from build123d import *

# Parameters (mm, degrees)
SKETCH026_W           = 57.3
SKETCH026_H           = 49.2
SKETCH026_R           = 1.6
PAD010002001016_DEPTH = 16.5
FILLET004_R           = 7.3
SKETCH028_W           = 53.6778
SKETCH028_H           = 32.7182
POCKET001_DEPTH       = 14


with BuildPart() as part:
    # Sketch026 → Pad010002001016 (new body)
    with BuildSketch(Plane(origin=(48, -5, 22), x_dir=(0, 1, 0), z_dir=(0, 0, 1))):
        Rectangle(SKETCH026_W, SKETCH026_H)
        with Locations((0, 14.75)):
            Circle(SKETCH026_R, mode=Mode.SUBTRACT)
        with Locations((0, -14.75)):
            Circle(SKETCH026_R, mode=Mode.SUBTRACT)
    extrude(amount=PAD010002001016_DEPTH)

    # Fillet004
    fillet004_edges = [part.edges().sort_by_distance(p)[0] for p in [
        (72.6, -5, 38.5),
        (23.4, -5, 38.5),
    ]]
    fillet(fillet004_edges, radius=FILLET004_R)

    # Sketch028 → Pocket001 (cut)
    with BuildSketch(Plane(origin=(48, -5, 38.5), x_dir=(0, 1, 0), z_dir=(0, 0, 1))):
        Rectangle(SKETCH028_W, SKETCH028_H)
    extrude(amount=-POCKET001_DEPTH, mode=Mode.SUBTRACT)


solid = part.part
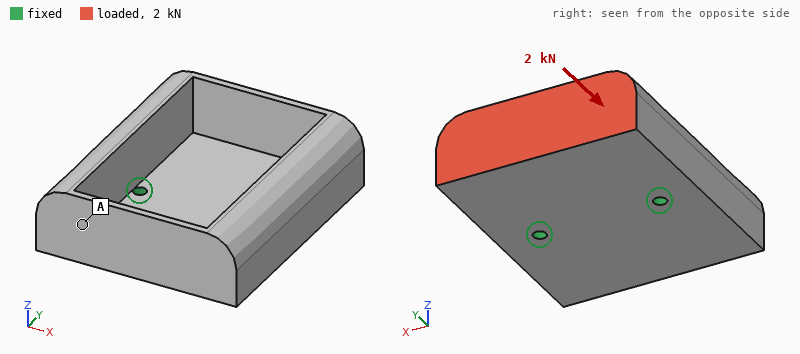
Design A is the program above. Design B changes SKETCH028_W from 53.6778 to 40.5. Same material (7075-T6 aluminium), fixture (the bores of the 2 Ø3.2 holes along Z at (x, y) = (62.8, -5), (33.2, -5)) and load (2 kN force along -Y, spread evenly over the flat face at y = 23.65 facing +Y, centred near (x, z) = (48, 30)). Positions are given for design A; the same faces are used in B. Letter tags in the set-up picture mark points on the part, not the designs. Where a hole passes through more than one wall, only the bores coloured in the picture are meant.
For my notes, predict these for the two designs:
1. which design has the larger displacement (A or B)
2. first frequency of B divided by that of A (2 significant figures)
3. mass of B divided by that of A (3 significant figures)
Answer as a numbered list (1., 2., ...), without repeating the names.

1. A
2. 0.81
3. 1.29
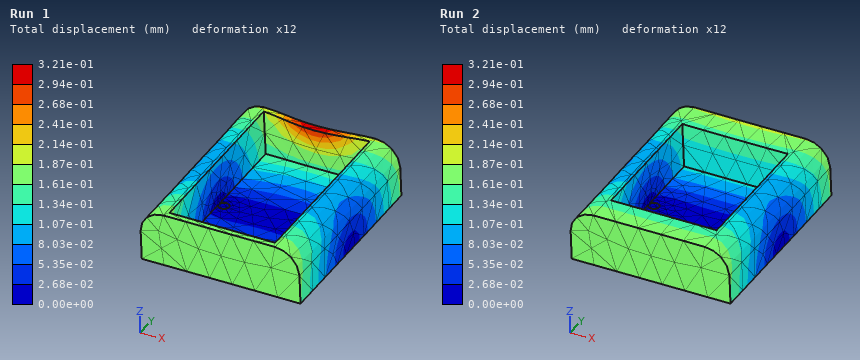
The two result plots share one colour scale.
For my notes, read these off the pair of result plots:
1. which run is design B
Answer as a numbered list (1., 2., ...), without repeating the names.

1. Run 2
